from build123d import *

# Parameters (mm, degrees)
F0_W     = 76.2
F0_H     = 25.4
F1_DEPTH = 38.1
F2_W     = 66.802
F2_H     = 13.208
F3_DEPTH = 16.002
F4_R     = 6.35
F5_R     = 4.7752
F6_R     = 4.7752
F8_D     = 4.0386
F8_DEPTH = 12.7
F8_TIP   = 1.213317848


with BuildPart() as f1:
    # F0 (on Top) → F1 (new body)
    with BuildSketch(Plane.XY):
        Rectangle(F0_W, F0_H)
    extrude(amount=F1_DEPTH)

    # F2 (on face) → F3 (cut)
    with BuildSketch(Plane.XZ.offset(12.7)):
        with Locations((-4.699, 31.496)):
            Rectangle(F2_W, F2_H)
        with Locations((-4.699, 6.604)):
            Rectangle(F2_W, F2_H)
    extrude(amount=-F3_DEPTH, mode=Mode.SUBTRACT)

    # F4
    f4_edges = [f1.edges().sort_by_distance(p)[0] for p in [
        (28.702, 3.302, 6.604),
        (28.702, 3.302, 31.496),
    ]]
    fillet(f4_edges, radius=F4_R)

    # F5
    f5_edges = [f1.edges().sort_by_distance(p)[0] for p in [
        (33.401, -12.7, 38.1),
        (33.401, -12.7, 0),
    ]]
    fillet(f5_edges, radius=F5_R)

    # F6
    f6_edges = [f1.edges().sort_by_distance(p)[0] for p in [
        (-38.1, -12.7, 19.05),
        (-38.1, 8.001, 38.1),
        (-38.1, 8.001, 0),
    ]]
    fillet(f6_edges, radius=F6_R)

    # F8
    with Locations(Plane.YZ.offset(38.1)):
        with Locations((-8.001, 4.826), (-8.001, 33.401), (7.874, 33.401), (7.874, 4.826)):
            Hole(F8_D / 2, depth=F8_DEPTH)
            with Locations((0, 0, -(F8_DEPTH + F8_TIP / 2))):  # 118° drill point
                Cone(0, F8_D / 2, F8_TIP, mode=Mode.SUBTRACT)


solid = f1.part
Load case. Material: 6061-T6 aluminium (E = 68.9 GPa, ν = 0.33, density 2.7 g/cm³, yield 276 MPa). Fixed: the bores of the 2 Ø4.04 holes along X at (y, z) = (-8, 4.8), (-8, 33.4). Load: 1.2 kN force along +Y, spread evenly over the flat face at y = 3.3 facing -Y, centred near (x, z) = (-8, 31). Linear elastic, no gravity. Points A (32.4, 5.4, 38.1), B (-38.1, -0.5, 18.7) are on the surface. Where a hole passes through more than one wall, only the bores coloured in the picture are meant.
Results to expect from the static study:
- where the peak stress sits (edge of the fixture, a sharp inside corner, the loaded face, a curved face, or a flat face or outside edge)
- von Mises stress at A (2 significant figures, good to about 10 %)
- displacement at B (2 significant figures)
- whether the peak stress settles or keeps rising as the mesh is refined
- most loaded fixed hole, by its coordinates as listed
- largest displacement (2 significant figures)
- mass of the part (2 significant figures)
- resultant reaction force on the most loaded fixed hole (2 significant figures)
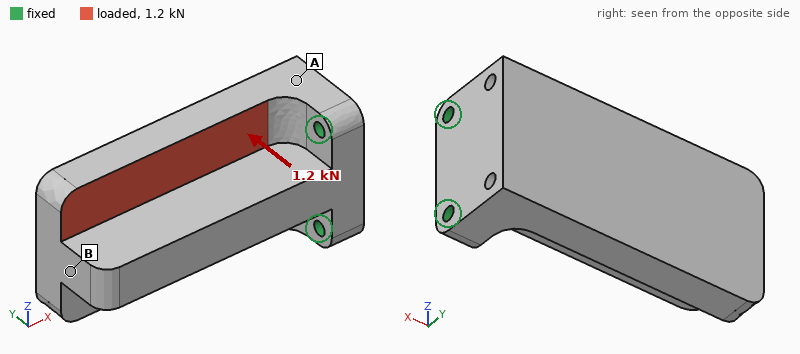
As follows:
edge of the fixture
31 MPa
0.23 mm
keeps rising
(-8, 33.4)
0.25 mm
120 g
1.2 kN
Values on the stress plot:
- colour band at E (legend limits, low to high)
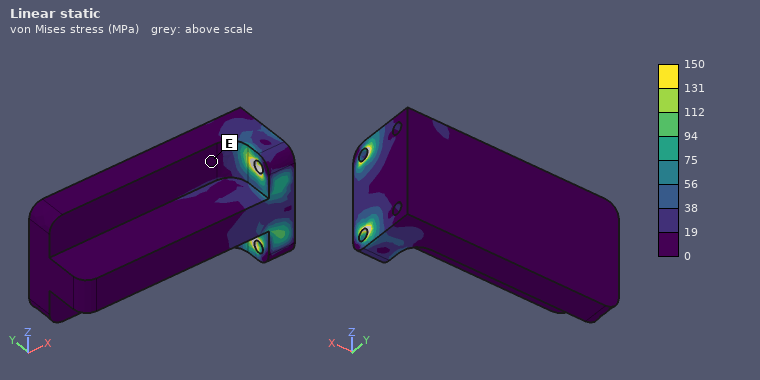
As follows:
0 to 19 MPa
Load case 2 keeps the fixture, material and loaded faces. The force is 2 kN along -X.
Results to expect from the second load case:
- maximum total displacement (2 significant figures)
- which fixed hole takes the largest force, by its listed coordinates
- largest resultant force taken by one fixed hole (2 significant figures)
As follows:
83 µm
(-8, 33.4)
1.9 kN
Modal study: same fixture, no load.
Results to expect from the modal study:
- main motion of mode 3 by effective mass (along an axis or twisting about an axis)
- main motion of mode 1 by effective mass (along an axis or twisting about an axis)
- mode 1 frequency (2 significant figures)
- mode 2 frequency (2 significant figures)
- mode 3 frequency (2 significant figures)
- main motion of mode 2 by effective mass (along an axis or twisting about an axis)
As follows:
twisting about X
along Y
1400 Hz
2600 Hz
6300 Hz
along Z
